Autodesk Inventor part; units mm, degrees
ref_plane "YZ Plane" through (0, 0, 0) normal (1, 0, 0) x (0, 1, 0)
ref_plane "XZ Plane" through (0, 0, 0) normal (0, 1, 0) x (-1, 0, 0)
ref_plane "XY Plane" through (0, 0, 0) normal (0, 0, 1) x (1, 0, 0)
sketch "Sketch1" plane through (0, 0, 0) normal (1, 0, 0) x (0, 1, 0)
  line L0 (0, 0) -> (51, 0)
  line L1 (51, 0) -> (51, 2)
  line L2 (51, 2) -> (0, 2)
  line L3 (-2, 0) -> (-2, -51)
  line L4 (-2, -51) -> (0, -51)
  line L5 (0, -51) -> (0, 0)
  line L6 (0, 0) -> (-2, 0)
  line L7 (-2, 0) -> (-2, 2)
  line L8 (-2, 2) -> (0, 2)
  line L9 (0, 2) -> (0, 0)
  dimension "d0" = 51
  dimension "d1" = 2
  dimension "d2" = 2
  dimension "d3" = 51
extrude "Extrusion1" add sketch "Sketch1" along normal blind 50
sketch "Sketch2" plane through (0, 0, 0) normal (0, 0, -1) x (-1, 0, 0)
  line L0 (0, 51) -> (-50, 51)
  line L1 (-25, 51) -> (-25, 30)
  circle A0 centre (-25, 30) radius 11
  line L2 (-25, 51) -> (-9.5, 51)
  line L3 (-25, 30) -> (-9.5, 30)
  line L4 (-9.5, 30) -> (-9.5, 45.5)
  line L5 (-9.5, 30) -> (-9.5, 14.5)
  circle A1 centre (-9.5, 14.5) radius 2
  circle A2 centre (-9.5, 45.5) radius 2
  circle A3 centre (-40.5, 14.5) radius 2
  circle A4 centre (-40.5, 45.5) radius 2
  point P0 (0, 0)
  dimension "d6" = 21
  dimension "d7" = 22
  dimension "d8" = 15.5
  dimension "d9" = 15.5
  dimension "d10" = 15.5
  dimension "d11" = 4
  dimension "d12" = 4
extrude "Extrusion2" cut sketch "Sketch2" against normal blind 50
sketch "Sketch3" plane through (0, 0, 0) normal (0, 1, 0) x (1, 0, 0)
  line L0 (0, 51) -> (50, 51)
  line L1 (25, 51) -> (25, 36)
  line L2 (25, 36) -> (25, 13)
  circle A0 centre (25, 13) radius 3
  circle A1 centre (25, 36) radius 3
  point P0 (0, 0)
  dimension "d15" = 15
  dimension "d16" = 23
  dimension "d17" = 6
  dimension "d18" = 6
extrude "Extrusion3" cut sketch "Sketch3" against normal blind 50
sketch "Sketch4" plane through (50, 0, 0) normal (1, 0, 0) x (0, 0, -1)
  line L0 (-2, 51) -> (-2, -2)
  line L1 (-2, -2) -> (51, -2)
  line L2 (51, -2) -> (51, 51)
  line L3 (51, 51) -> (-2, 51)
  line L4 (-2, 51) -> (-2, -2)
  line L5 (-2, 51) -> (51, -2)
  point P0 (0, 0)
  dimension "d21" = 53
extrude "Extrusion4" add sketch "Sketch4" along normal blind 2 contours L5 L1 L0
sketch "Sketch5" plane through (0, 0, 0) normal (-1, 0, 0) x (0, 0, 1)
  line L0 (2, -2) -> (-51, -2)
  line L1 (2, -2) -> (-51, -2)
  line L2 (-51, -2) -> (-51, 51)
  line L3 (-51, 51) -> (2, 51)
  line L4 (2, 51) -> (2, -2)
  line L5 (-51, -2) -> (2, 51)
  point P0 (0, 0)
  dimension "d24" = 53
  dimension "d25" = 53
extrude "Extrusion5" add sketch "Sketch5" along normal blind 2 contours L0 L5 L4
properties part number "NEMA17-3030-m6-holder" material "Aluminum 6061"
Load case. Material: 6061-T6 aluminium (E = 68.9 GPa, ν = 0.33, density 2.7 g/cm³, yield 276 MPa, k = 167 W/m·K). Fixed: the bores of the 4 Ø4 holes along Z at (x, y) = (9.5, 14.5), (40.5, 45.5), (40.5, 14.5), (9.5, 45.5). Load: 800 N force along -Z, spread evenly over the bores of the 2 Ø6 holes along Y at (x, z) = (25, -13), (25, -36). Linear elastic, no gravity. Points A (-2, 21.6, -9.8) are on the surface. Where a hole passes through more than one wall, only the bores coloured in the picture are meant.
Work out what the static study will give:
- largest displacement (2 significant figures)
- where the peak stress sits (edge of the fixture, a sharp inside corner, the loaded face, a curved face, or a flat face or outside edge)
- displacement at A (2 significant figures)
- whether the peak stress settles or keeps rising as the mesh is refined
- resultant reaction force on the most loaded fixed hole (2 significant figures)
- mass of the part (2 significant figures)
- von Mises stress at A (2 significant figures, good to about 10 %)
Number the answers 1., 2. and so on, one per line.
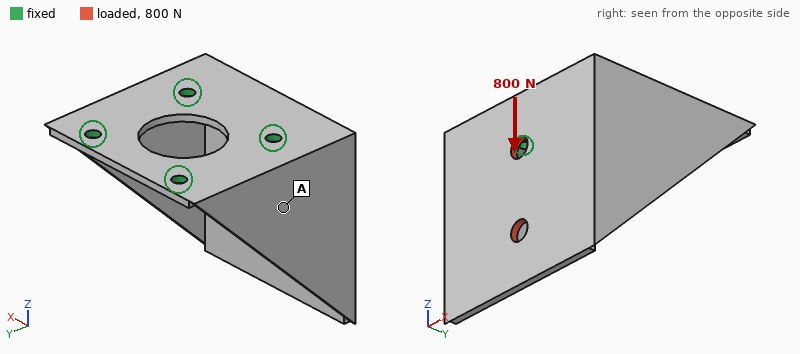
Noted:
1. 0.21 mm
2. edge of the fixture
3. 0.049 mm
4. keeps rising
5. 550 N
6. 41 g
7. 16 MPa
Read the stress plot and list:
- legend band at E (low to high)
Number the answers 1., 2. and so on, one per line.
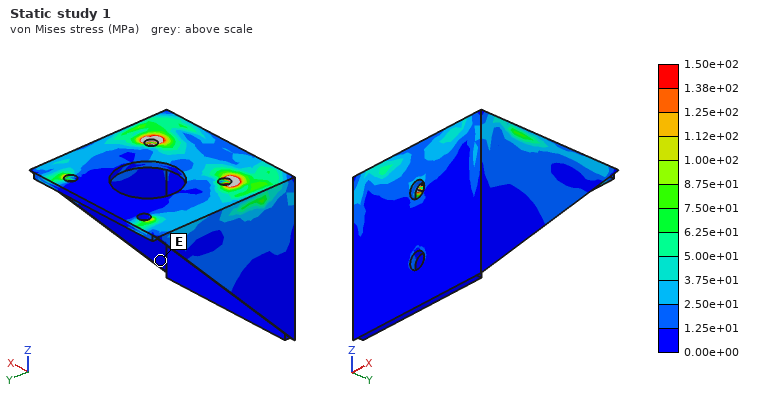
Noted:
1. 0.00e+00 to 1.25e+01 MPa
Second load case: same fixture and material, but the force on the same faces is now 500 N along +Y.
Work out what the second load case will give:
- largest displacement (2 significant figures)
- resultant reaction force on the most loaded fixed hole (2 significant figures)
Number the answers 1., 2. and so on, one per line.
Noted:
1. 0.51 mm
2. 290 N
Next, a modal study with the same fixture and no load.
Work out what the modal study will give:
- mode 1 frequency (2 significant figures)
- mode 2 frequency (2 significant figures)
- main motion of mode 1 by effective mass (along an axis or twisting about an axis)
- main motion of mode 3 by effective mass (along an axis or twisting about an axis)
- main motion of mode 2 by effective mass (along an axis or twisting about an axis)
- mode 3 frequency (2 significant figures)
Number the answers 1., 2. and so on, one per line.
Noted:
1. 1500 Hz
2. 1700 Hz
3. along X
4. along Z
5. along Y
6. 2900 Hz
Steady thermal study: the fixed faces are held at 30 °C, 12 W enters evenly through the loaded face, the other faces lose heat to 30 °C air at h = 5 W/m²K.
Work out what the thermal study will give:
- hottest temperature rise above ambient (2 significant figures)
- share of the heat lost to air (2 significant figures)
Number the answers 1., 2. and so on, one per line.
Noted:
1. 21 K
2. 5.3 %
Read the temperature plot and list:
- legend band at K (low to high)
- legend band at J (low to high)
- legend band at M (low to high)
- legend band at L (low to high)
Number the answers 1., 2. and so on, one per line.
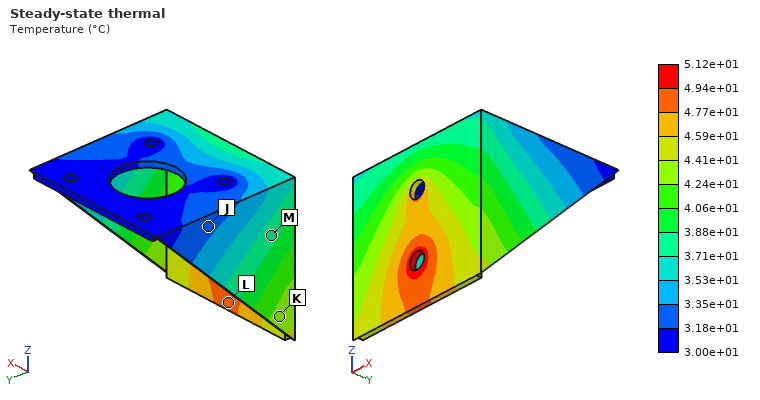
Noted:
1. 4.24e+01 to 4.41e+01 °C
2. 3.18e+01 to 3.35e+01 °C
3. 3.71e+01 to 3.88e+01 °C
4. 4.77e+01 to 4.94e+01 °C
